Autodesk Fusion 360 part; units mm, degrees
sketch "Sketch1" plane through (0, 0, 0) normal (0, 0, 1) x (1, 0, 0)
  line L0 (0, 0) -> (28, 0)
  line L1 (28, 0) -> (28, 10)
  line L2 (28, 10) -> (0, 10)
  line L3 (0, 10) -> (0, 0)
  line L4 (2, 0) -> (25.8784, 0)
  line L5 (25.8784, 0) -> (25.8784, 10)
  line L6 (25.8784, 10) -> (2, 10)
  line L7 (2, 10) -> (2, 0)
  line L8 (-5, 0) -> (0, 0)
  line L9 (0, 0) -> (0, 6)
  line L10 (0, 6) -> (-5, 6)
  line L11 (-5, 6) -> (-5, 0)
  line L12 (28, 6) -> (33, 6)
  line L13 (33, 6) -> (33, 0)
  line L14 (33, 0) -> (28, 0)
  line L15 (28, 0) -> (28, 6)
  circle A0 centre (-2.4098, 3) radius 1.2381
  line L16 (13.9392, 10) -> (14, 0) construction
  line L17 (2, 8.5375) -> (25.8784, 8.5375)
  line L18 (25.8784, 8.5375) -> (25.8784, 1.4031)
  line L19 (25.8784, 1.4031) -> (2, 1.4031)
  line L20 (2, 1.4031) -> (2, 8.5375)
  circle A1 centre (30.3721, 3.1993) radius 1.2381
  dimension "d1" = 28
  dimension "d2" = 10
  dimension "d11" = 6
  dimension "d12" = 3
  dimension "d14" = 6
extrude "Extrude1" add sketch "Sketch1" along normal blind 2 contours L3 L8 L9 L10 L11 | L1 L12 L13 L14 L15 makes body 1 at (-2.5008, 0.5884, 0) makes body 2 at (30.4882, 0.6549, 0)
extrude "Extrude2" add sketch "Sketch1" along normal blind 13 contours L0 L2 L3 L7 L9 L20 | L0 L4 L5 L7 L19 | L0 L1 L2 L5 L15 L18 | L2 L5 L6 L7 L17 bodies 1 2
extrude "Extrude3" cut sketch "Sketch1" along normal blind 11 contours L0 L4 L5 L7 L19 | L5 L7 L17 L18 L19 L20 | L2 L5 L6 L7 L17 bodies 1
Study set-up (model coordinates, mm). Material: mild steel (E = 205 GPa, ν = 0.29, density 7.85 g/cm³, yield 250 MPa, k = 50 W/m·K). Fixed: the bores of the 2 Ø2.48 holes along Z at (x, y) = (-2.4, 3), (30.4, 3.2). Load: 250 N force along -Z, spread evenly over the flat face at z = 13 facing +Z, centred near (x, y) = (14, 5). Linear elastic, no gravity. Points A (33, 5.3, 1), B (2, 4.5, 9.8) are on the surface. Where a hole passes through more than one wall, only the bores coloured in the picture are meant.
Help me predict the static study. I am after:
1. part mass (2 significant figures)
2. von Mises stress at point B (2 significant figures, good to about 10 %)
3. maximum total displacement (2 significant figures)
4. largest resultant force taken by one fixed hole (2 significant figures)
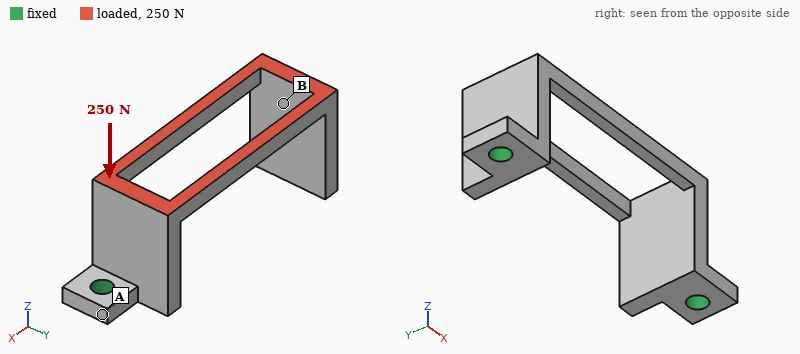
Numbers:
6.1 g
31 MPa
29 µm
140 N
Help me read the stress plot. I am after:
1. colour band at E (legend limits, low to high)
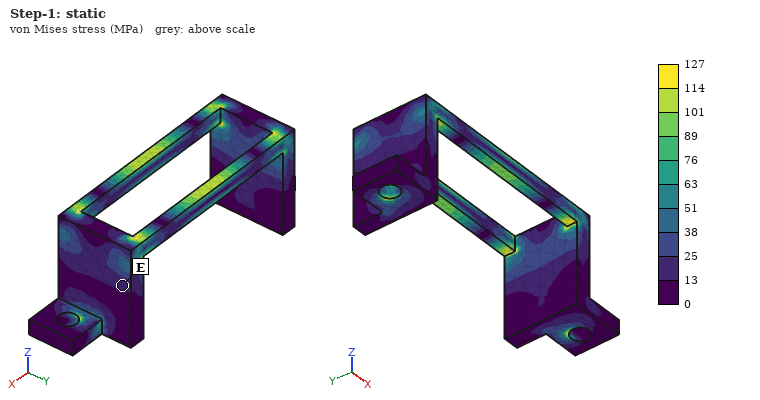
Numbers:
13 to 25 MPa
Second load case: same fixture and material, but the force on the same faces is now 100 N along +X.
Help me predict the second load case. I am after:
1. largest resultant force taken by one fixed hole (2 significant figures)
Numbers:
54 N
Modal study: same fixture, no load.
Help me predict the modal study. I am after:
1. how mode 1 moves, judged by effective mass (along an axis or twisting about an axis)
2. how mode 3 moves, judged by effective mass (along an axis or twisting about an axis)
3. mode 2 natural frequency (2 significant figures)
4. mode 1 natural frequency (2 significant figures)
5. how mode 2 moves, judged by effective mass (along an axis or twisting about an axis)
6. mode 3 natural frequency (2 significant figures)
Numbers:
along X
twisting about Z
7500 Hz
7000 Hz
along Y
9700 Hz
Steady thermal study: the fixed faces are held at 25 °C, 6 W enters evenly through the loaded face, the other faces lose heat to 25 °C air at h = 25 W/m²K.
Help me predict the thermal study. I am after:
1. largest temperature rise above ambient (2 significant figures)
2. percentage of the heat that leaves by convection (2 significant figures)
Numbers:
79 K
14 %
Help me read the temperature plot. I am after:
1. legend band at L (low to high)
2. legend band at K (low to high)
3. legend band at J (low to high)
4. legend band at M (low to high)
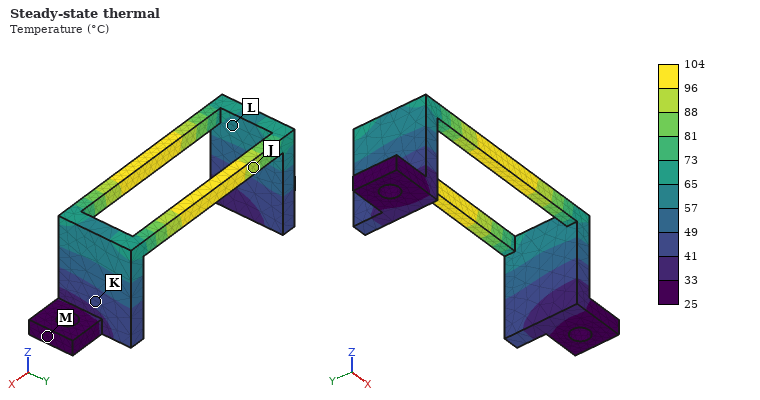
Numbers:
57 to 65 °C
41 to 49 °C
88 to 96 °C
25 to 33 °C
